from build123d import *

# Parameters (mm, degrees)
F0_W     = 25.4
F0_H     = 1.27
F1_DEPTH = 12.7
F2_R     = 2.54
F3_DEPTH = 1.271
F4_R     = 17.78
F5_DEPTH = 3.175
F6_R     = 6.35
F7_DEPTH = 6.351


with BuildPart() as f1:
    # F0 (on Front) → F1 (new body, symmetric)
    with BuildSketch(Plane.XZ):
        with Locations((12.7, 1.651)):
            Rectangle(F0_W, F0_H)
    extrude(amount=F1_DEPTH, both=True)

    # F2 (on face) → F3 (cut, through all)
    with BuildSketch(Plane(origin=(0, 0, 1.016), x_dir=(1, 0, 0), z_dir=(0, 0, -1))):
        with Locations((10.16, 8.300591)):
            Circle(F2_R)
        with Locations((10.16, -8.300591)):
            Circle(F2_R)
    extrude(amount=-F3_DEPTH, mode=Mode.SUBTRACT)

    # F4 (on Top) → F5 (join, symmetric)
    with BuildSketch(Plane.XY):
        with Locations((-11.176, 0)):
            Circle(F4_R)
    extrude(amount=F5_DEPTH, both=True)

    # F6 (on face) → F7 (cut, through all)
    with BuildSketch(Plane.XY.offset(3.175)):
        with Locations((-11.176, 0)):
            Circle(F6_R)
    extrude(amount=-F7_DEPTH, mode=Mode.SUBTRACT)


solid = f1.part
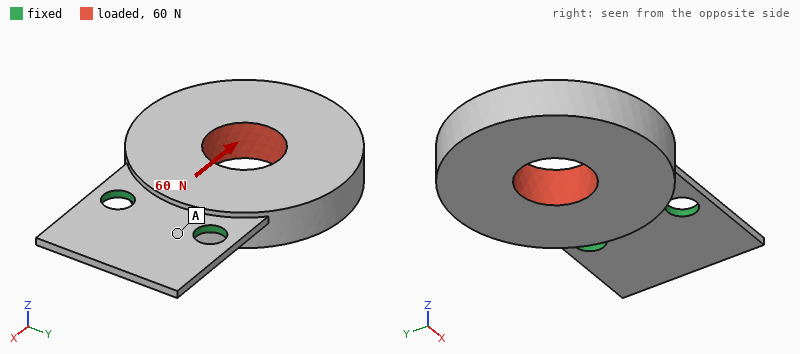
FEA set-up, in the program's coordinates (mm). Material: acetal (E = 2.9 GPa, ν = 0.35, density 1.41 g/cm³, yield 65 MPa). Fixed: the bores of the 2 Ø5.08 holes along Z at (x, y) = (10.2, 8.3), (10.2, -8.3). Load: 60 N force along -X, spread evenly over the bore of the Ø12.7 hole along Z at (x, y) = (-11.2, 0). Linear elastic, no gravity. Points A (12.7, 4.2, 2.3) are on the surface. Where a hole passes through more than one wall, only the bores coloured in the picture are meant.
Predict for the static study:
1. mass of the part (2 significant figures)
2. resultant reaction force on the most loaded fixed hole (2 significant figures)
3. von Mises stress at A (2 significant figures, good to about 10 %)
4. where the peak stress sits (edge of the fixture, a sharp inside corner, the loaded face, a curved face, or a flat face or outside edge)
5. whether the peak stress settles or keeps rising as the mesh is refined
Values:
8.6 g
30 N
2.0 MPa
edge of the fixture
keeps rising
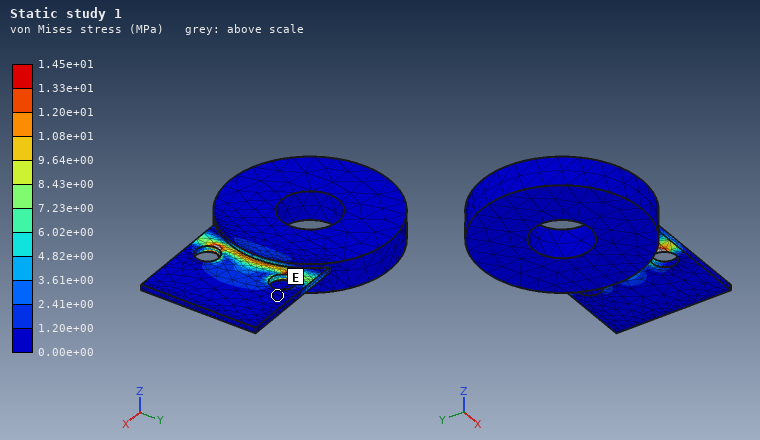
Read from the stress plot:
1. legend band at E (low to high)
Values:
0.00e+00 to 1.20e+00 MPa
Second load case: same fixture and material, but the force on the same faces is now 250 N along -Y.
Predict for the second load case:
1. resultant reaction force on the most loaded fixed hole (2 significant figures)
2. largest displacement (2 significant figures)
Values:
310 N
0.31 mm
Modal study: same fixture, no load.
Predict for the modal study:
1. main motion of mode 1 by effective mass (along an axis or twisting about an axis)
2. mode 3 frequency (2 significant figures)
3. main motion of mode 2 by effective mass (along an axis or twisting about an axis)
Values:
along Z
1600 Hz
twisting about X
